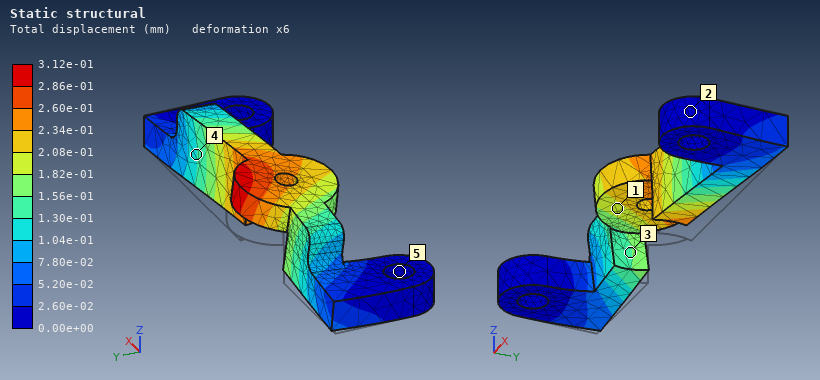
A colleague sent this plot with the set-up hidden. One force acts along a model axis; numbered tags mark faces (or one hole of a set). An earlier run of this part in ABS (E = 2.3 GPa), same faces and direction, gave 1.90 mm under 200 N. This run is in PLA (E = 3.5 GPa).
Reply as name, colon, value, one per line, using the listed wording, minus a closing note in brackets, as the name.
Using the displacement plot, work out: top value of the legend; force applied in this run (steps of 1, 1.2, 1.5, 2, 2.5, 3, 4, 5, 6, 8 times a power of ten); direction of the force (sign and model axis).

top value of the legend: 3.12e-01 mm
force applied in this run: 50 N
direction of the force: +Z
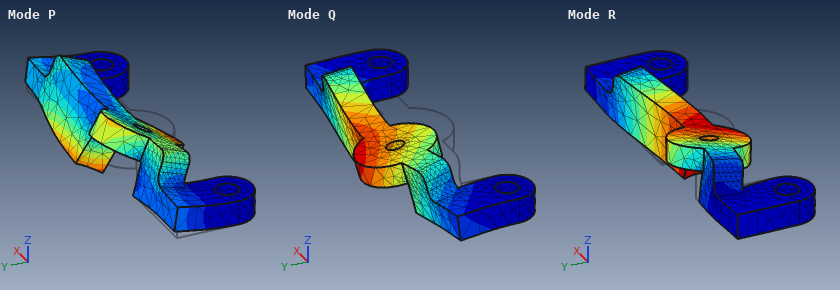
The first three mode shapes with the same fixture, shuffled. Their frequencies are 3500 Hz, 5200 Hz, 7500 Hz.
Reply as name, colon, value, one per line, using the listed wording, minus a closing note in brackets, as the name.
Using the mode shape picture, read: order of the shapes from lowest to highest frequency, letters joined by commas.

order of the shapes from lowest to highest frequency, letters joined by commas: Q, R, P
